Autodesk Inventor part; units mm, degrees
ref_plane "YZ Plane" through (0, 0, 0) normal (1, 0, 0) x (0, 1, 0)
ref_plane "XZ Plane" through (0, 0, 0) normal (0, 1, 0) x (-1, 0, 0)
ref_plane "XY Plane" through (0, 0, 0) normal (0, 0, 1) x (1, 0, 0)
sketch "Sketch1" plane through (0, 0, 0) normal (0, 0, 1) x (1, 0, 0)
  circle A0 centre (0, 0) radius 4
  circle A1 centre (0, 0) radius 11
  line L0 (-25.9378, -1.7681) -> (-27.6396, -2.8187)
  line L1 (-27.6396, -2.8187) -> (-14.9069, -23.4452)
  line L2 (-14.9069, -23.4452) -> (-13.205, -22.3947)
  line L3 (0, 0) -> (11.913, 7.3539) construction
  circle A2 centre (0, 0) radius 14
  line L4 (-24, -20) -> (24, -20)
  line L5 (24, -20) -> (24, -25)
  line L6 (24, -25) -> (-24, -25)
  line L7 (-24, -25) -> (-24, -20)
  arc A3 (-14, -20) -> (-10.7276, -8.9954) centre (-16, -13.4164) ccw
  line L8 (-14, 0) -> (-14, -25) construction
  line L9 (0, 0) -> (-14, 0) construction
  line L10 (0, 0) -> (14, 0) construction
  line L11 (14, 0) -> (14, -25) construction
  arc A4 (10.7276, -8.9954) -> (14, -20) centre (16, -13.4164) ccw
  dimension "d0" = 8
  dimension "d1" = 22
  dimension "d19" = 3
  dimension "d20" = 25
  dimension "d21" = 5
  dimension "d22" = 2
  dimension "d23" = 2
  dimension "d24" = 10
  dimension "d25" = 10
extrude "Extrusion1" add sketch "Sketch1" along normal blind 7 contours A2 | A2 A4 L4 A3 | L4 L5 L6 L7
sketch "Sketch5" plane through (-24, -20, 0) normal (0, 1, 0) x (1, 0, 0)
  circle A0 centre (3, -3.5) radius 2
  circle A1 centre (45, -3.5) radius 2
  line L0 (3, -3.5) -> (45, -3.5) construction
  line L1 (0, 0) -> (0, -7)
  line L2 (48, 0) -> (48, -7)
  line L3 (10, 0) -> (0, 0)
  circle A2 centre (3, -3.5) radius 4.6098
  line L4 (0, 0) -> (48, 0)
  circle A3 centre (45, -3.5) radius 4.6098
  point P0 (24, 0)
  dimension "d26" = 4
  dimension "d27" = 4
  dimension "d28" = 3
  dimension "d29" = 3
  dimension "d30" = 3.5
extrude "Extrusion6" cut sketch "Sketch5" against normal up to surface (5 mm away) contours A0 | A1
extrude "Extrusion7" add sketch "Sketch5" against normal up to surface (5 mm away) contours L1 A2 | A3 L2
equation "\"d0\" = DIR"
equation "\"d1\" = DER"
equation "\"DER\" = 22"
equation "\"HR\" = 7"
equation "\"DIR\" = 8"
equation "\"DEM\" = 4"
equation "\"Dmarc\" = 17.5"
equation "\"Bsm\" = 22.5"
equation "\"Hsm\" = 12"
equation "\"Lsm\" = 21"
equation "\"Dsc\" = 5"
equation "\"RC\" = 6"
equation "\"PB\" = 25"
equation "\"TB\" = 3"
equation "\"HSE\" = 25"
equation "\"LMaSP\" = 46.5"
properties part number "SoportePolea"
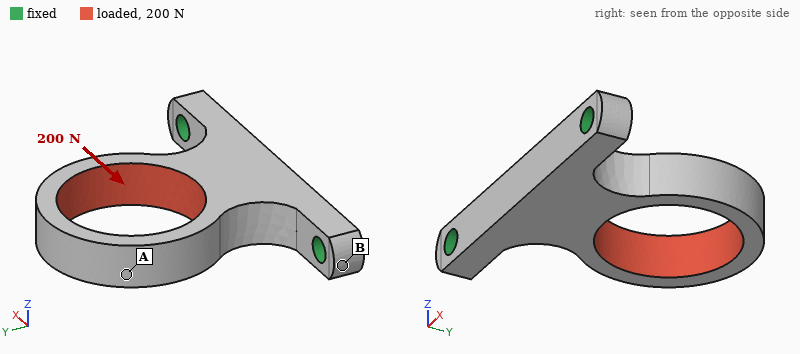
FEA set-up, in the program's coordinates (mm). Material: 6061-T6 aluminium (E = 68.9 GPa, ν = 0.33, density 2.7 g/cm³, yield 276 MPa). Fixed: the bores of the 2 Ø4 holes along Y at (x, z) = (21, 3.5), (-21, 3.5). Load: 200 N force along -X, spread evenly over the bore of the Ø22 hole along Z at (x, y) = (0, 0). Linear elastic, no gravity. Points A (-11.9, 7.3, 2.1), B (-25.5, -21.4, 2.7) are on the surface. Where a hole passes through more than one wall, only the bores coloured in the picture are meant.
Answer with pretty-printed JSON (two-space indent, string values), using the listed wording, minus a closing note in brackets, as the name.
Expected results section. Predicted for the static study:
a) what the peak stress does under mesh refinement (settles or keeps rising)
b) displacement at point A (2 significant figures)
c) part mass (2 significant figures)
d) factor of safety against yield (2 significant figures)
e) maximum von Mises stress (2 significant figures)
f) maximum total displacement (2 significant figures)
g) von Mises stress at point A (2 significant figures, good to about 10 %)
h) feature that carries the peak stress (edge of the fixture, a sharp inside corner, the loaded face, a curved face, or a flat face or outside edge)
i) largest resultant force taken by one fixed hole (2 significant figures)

{
  "what the peak stress does under mesh refinement": "settles",
  "displacement at point A": "63 µm",
  "part mass": "12 g",
  "factor of safety against yield": "5.1",
  "maximum von Mises stress": "54 MPa",
  "maximum total displacement": "69 µm",
  "von Mises stress at point A": "22 MPa",
  "feature that carries the peak stress": "the loaded face",
  "largest resultant force taken by one fixed hole": "170 N"
}
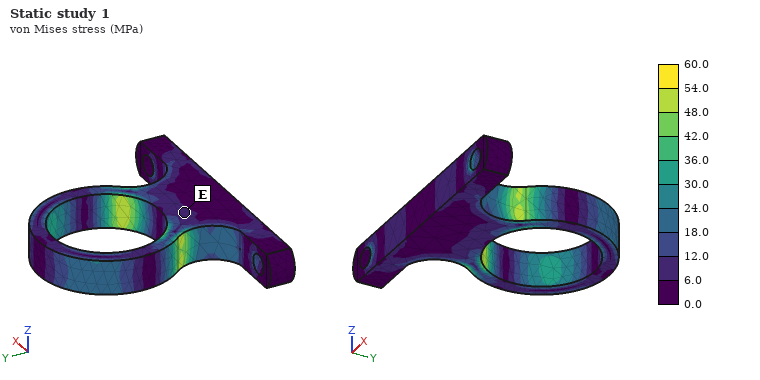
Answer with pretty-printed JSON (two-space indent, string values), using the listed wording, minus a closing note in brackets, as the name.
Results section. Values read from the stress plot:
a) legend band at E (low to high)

{
  "legend band at E": "6.0 to 12.0 MPa"
}
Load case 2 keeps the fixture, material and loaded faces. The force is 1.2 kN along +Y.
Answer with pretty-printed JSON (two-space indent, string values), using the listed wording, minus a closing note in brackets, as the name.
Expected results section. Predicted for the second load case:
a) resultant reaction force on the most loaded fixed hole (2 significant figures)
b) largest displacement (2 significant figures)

{
  "resultant reaction force on the most loaded fixed hole": "700 N",
  "largest displacement": "70 µm"
}
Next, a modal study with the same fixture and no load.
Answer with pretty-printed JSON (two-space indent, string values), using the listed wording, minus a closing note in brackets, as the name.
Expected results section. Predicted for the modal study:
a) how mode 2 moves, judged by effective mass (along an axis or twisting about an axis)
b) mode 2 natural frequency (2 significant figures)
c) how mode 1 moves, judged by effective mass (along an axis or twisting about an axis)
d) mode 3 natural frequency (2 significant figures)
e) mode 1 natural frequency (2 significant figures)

{
  "how mode 2 moves, judged by effective mass": "along X",
  "mode 2 natural frequency": "4400 Hz",
  "how mode 1 moves, judged by effective mass": "along Z",
  "mode 3 natural frequency": "8800 Hz",
  "mode 1 natural frequency": "2400 Hz"
}
